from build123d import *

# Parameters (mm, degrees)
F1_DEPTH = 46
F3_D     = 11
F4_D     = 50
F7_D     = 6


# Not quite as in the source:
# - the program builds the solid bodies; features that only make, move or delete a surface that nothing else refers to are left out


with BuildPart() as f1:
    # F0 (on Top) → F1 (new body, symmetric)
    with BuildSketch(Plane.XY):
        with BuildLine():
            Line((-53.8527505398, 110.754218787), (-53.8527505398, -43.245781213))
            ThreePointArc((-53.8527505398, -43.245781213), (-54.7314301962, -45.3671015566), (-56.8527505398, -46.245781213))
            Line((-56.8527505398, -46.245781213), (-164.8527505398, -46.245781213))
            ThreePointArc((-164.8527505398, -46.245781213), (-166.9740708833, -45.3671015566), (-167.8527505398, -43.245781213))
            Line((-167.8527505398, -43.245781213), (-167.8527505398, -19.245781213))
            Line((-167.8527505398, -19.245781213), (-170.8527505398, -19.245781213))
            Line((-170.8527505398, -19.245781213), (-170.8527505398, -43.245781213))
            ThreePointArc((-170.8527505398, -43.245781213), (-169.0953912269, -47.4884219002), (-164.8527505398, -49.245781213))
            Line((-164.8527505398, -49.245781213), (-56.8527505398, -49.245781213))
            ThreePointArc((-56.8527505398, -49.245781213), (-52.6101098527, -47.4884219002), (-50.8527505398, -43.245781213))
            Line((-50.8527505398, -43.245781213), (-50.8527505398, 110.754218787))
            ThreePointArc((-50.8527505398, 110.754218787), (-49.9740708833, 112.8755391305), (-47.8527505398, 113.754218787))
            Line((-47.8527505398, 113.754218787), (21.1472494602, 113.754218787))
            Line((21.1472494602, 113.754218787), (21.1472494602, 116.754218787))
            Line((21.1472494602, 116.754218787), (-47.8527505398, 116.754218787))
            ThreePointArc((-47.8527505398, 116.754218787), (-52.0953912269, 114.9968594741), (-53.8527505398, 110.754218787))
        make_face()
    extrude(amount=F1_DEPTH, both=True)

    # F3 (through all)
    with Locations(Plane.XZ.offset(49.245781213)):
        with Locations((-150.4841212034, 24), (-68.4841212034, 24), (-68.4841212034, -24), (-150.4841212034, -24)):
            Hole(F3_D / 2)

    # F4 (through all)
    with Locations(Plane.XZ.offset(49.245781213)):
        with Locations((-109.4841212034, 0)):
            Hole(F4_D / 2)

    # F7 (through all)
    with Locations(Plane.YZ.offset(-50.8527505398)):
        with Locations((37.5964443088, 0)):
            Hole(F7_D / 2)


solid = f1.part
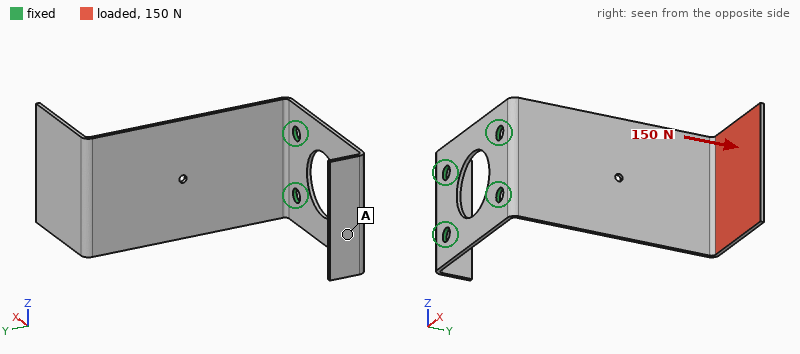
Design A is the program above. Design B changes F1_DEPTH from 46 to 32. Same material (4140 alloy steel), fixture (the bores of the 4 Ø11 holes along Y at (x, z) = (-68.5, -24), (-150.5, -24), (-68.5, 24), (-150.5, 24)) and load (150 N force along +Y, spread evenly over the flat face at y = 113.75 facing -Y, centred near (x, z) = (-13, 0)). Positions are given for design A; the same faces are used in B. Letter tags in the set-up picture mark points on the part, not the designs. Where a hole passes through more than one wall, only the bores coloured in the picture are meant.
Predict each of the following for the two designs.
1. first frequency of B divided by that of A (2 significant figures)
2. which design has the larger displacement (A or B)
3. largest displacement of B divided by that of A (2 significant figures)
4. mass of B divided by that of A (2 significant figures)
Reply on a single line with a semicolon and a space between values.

1.0; B; 1.4; 0.67
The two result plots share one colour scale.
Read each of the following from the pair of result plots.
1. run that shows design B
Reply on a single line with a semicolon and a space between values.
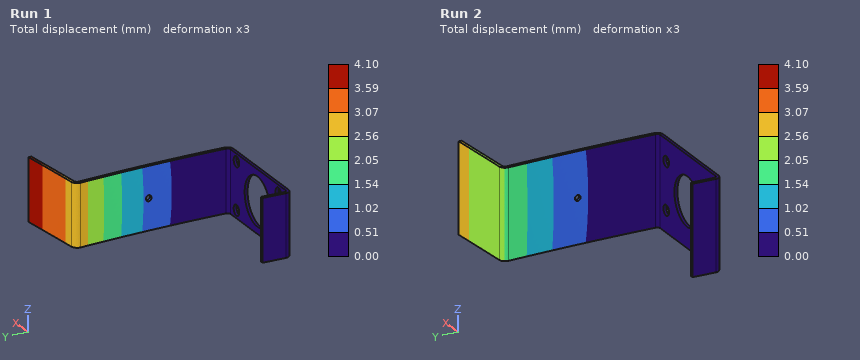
Run 1
